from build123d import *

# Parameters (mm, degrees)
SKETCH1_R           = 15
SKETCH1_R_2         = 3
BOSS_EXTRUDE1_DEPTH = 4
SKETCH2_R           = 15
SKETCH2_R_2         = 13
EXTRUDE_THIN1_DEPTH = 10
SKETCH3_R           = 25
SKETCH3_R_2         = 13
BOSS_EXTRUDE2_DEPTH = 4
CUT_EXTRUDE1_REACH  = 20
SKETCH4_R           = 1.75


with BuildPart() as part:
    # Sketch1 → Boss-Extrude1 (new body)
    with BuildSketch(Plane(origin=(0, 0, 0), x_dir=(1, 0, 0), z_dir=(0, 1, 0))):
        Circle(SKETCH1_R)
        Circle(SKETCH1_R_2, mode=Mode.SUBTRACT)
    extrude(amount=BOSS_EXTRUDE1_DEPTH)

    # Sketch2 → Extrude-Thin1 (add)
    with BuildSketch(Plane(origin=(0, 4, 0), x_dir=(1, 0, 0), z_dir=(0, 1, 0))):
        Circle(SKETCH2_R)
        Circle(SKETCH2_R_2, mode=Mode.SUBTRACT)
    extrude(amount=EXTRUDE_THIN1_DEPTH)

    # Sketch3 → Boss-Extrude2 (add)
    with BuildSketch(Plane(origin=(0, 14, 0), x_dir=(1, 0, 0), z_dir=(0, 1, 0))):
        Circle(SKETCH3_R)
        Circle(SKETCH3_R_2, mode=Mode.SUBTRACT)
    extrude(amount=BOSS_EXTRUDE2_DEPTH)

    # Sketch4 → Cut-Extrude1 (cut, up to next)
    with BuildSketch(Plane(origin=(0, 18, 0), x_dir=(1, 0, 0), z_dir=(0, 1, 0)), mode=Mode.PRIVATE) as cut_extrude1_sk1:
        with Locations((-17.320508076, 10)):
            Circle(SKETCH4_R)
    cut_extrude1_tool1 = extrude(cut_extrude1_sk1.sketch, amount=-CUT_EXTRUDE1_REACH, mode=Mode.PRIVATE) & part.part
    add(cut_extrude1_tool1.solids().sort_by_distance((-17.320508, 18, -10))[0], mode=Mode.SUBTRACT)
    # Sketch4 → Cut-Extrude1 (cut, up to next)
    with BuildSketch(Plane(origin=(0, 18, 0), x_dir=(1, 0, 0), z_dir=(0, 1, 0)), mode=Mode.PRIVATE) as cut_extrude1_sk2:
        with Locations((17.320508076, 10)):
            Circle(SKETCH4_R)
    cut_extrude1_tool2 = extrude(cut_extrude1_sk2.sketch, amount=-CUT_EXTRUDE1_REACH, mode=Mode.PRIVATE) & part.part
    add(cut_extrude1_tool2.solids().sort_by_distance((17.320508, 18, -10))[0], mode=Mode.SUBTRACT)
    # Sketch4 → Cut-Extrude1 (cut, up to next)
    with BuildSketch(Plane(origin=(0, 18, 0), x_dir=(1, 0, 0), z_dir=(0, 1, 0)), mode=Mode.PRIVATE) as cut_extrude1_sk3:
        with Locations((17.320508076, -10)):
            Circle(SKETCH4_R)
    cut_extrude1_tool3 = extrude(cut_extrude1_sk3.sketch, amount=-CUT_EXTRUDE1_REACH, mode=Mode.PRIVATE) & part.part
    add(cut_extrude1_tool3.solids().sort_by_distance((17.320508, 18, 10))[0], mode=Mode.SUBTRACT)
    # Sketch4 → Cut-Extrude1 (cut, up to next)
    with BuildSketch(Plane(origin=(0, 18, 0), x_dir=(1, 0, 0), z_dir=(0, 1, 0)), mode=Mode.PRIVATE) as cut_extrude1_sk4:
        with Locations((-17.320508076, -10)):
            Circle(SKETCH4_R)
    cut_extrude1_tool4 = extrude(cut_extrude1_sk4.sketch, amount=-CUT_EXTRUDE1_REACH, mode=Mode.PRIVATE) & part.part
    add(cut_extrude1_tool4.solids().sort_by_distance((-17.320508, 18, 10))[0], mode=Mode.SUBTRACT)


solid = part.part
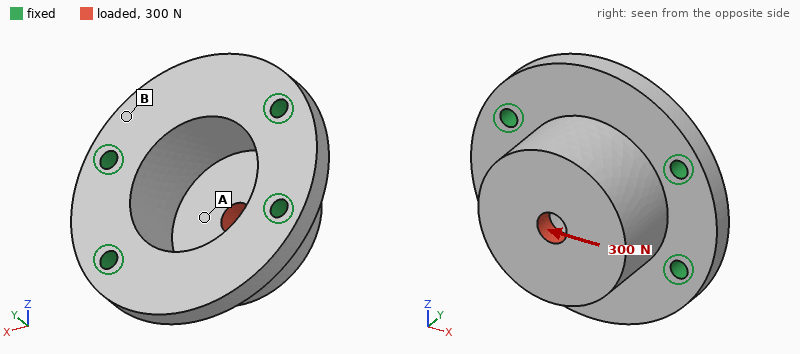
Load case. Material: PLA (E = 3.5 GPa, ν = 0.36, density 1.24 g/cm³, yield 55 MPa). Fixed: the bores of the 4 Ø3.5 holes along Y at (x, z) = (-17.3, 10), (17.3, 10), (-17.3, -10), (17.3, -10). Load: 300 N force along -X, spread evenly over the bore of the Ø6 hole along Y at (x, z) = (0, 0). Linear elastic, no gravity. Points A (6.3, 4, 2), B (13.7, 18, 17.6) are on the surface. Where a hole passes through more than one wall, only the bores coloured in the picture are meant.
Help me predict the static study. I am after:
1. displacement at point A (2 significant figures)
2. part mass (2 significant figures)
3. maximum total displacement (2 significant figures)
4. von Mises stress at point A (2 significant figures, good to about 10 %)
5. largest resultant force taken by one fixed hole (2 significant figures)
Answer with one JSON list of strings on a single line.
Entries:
["61 µm", "12 g", "70 µm", "3.8 MPa", "100 N"]
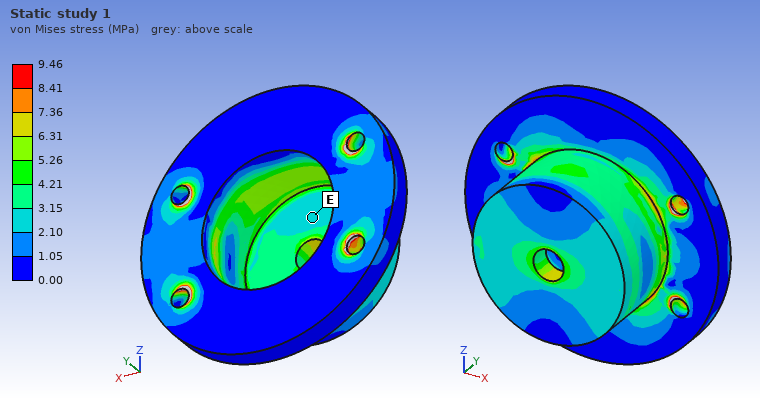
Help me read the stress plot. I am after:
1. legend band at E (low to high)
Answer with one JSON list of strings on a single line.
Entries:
["2.10 to 3.15 MPa"]
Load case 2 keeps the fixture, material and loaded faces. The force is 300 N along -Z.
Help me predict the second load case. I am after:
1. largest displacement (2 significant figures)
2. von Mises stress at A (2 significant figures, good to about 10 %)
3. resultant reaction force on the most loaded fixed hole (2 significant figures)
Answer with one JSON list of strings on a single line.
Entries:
["0.12 mm", "2.7 MPa", "130 N"]
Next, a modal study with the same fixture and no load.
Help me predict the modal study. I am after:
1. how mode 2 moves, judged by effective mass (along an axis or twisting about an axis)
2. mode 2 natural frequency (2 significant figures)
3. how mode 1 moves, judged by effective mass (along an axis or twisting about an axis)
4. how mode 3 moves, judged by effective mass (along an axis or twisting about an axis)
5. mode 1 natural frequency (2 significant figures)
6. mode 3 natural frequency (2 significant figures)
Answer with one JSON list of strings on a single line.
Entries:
["along Y", "4800 Hz", "along Z", "along X", "3500 Hz", "5600 Hz"]
